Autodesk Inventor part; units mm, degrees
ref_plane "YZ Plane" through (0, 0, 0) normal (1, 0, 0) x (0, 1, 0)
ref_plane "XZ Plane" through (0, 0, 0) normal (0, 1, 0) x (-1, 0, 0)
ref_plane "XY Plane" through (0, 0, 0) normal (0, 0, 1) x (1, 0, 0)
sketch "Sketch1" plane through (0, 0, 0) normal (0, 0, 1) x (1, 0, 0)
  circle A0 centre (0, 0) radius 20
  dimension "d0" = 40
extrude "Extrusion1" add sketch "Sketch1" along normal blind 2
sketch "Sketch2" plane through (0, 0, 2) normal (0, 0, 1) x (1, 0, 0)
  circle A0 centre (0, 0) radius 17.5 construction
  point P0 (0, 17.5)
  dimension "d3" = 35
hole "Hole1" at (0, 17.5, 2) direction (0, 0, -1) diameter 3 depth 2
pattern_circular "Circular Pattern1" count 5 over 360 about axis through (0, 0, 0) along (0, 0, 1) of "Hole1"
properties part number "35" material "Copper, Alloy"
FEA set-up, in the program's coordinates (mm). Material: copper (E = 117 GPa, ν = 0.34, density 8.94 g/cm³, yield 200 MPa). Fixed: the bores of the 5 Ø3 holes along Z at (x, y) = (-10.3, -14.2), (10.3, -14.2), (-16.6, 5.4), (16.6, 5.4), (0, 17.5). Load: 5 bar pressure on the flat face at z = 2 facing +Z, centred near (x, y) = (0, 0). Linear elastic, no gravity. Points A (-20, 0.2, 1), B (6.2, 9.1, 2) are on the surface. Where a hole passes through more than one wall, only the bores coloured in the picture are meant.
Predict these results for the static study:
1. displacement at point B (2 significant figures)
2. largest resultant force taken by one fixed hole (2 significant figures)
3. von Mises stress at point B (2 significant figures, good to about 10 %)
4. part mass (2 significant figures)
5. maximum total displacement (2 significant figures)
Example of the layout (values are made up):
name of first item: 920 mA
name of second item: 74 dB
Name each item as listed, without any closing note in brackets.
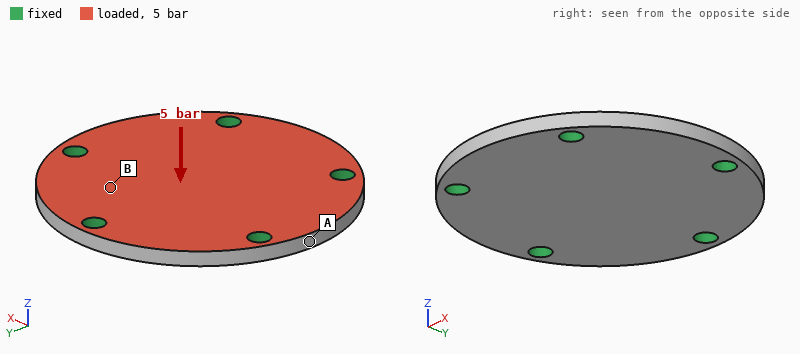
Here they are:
displacement at point B: 5.3 µm
largest resultant force taken by one fixed hole: 120 N
von Mises stress at point B: 16 MPa
part mass: 22 g
maximum total displacement: 10 µm
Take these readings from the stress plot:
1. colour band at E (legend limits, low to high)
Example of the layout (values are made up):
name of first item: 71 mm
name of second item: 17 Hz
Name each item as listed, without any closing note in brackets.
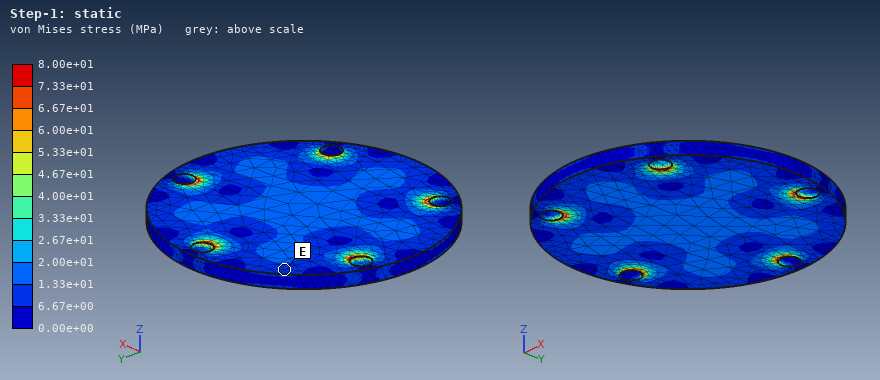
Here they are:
colour band at E: 6.67e+00 to 1.33e+01 MPa
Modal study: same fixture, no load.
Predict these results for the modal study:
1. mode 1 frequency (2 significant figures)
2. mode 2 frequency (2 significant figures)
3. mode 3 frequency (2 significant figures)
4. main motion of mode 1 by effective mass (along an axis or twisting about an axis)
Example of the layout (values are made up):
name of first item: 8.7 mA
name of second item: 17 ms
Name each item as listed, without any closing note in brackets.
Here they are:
mode 1 frequency: 10 kHz
mode 2 frequency: 17 kHz
mode 3 frequency: 17 kHz
main motion of mode 1 by effective mass: along Z
